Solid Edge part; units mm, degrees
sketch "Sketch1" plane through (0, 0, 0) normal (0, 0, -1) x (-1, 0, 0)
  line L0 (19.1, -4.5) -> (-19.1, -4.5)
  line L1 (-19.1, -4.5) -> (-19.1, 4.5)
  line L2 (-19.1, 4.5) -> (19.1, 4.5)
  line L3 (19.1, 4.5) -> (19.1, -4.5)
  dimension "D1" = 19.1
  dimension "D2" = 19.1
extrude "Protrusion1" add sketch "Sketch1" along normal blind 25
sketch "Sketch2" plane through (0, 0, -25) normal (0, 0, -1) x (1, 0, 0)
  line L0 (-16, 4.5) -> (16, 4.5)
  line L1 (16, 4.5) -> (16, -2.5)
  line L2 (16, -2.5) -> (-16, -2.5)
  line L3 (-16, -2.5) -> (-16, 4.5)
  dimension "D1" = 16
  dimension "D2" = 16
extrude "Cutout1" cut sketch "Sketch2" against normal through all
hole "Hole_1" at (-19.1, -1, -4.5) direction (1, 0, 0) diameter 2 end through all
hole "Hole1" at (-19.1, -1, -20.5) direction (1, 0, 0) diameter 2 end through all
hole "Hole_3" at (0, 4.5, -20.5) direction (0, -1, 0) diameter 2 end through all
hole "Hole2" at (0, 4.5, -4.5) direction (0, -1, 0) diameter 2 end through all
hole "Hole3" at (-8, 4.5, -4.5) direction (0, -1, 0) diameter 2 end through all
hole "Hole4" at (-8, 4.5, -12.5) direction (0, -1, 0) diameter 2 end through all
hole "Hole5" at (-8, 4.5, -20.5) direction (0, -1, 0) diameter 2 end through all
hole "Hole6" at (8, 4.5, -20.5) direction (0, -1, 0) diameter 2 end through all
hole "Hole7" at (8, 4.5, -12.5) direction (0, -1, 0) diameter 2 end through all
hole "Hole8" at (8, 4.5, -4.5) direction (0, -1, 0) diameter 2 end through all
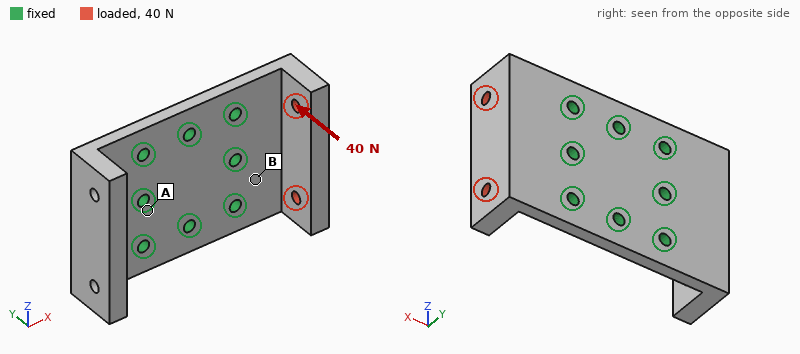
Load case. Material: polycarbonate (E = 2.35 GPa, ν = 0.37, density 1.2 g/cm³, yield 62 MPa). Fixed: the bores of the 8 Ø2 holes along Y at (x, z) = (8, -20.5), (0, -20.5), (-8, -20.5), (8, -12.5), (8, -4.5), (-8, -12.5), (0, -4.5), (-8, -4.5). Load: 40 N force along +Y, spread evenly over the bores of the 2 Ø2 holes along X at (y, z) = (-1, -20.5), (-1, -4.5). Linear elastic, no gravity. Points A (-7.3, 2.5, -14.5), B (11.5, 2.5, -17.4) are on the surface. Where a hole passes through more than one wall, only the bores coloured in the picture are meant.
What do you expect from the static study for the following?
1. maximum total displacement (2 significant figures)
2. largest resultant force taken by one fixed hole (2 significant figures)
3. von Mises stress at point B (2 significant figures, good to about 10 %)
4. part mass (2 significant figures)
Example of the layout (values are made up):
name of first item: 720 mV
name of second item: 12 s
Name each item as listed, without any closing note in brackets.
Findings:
maximum total displacement: 0.47 mm
largest resultant force taken by one fixed hole: 17 N
von Mises stress at point B: 12 MPa
part mass: 3.5 g
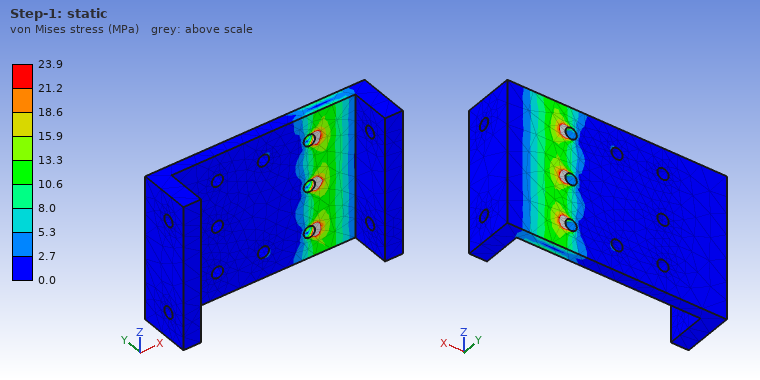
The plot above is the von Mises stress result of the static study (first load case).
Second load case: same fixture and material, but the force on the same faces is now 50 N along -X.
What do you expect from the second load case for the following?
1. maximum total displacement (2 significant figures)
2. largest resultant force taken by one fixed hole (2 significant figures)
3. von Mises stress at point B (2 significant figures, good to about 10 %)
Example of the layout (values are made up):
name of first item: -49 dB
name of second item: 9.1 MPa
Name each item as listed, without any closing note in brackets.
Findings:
maximum total displacement: 0.49 mm
largest resultant force taken by one fixed hole: 15 N
von Mises stress at point B: 12 MPa
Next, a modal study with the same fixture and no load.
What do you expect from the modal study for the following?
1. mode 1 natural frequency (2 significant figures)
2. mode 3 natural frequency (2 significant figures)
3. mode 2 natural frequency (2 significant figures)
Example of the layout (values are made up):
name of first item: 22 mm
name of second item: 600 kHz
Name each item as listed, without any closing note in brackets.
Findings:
mode 1 natural frequency: 1700 Hz
mode 3 natural frequency: 3100 Hz
mode 2 natural frequency: 1700 Hz
